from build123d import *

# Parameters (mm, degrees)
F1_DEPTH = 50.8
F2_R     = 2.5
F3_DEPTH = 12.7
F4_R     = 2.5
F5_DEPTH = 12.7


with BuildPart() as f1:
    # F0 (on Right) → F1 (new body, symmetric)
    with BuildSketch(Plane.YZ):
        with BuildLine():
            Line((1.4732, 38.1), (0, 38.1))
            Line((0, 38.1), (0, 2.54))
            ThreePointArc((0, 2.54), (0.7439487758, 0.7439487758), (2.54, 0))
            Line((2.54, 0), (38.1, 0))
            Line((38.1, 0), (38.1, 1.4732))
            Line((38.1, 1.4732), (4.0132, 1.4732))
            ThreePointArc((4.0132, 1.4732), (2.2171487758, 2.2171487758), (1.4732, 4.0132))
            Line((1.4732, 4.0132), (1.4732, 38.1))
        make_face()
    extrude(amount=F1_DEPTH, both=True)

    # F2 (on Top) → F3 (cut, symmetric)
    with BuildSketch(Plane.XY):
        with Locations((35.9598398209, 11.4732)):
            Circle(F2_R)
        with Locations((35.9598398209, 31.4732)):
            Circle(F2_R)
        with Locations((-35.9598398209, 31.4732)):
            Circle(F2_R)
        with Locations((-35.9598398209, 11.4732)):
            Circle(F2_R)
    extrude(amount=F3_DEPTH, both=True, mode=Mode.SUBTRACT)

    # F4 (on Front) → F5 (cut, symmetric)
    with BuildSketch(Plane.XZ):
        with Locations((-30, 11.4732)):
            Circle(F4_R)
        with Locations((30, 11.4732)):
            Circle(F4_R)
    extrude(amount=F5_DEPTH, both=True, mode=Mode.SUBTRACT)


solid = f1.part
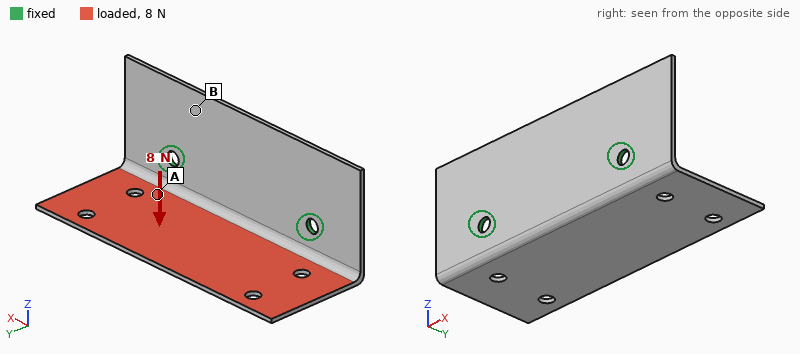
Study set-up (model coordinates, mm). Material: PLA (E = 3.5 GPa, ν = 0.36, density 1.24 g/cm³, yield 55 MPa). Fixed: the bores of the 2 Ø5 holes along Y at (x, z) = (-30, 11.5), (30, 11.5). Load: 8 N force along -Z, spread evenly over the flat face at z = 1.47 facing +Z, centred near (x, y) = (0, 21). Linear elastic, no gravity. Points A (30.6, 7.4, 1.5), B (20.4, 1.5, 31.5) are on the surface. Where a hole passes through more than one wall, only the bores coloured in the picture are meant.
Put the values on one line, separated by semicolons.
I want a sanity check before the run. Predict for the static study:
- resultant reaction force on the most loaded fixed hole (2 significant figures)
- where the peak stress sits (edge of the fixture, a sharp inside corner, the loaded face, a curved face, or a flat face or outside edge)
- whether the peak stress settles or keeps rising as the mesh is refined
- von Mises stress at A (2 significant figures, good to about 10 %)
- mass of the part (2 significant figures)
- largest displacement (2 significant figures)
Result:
4.0 N; edge of the fixture; keeps rising; 2.6 MPa; 14 g; 1.1 mm
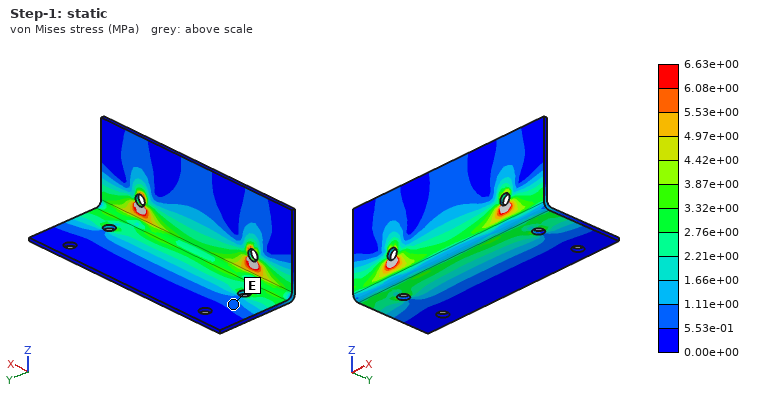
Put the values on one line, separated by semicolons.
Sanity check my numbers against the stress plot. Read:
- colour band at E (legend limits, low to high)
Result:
5.53e-01 to 1.11e+00 MPa
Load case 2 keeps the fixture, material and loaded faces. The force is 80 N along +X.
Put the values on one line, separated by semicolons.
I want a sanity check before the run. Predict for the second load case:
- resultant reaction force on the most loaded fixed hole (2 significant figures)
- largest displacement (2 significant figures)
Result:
49 N; 1.2 mm
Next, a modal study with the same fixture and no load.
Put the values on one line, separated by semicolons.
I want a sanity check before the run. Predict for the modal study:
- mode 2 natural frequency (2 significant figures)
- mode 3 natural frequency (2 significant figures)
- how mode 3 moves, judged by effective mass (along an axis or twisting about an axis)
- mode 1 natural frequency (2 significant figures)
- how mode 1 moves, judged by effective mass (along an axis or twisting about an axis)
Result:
310 Hz; 490 Hz; along Y; 210 Hz; along Z
